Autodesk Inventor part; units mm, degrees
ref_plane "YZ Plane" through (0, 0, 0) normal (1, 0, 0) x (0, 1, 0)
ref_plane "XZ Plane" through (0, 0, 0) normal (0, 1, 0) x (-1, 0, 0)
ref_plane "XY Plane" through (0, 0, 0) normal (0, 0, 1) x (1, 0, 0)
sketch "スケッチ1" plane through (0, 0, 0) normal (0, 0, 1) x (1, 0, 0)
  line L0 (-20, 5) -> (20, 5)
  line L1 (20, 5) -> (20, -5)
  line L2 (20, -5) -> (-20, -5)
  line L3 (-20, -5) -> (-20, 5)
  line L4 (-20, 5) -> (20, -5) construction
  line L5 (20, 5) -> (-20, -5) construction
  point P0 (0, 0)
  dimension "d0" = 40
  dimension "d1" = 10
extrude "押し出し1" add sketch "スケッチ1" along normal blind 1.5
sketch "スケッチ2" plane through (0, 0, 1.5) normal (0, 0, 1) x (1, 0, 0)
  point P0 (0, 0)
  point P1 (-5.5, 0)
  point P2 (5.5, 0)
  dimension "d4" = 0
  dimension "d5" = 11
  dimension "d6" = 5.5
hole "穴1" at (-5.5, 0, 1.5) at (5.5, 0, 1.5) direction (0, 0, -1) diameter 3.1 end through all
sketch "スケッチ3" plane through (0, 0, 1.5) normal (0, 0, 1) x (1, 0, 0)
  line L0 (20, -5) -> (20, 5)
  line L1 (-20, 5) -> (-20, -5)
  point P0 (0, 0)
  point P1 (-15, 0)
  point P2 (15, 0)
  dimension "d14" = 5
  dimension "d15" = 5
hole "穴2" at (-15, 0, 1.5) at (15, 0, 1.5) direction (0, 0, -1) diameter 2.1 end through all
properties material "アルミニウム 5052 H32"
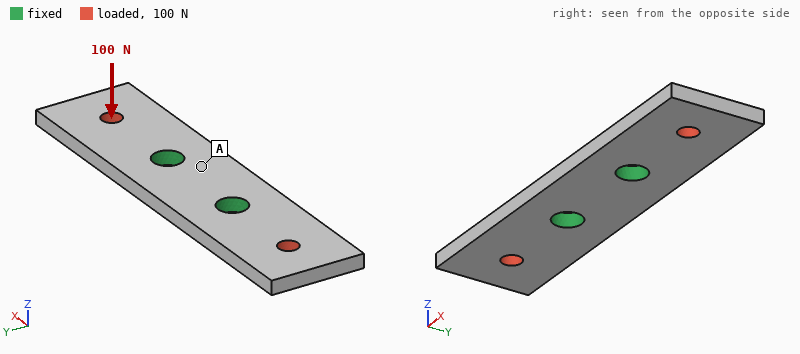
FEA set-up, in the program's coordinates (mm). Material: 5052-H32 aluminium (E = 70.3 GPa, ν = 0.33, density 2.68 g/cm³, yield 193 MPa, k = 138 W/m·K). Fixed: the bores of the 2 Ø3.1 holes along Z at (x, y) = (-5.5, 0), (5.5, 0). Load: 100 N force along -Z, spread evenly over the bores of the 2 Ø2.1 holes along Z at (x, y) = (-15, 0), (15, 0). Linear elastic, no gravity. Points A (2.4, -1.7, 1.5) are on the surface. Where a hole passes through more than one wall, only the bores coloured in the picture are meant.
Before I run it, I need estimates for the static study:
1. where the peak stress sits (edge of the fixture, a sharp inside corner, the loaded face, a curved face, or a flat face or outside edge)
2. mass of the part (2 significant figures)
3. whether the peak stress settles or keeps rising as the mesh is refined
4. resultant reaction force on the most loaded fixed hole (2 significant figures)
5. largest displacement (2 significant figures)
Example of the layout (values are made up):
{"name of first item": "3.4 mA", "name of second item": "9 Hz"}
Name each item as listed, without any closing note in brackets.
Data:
{"where the peak stress sits": "edge of the fixture", "mass of the part": "1.5 g", "whether the peak stress settles or keeps rising as the mesh is refined": "keeps rising", "resultant reaction force on the most loaded fixed hole": "50 N", "largest displacement": "0.10 mm"}
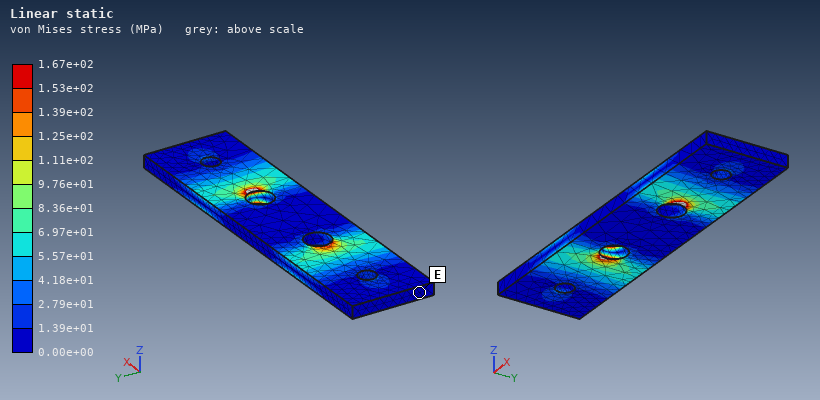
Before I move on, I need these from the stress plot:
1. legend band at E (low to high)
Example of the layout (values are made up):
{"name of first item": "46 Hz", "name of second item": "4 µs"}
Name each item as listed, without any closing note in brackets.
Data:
{"legend band at E": "0.00e+00 to 1.39e+01 MPa"}
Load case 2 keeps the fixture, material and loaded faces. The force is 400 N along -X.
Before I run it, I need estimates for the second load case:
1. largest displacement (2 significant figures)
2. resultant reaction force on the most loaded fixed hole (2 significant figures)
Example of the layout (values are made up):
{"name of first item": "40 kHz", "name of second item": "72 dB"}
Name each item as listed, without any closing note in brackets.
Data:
{"largest displacement": "2.9 µm", "resultant reaction force on the most loaded fixed hole": "200 N"}
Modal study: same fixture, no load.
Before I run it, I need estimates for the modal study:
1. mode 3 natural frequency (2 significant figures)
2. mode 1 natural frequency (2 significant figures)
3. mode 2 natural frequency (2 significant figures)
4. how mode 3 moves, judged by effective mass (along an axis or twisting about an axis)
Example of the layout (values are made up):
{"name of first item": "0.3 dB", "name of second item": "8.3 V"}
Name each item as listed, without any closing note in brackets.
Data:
{"mode 3 natural frequency": "17 kHz", "mode 1 natural frequency": "6800 Hz", "mode 2 natural frequency": "6800 Hz", "how mode 3 moves, judged by effective mass": "twisting about X"}
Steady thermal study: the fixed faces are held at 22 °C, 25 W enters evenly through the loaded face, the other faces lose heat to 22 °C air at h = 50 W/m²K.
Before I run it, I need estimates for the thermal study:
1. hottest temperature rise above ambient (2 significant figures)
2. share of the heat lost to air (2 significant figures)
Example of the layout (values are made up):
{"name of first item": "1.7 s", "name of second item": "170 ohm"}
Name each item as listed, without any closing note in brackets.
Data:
{"hottest temperature rise above ambient": "64 K", "share of the heat lost to air": "5.1 %"}
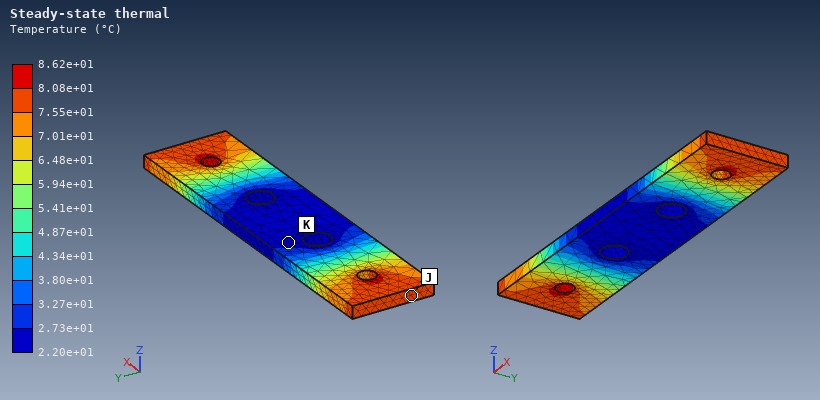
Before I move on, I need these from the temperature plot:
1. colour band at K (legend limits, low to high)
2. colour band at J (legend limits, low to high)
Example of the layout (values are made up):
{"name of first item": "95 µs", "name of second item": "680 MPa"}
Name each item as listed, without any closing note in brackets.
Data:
{"colour band at K": "2.20e+01 to 2.73e+01 °C", "colour band at J": "7.55e+01 to 8.08e+01 °C"}
